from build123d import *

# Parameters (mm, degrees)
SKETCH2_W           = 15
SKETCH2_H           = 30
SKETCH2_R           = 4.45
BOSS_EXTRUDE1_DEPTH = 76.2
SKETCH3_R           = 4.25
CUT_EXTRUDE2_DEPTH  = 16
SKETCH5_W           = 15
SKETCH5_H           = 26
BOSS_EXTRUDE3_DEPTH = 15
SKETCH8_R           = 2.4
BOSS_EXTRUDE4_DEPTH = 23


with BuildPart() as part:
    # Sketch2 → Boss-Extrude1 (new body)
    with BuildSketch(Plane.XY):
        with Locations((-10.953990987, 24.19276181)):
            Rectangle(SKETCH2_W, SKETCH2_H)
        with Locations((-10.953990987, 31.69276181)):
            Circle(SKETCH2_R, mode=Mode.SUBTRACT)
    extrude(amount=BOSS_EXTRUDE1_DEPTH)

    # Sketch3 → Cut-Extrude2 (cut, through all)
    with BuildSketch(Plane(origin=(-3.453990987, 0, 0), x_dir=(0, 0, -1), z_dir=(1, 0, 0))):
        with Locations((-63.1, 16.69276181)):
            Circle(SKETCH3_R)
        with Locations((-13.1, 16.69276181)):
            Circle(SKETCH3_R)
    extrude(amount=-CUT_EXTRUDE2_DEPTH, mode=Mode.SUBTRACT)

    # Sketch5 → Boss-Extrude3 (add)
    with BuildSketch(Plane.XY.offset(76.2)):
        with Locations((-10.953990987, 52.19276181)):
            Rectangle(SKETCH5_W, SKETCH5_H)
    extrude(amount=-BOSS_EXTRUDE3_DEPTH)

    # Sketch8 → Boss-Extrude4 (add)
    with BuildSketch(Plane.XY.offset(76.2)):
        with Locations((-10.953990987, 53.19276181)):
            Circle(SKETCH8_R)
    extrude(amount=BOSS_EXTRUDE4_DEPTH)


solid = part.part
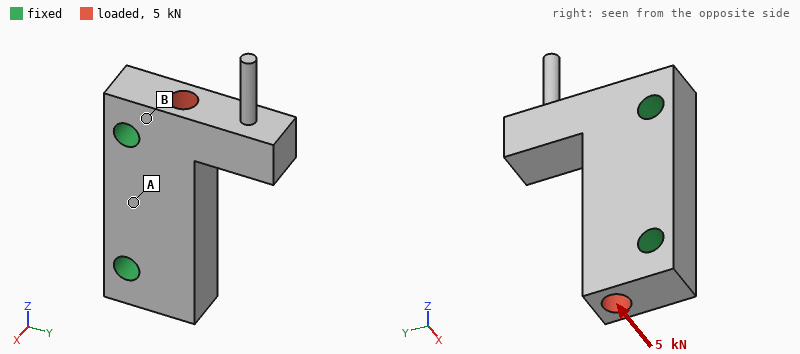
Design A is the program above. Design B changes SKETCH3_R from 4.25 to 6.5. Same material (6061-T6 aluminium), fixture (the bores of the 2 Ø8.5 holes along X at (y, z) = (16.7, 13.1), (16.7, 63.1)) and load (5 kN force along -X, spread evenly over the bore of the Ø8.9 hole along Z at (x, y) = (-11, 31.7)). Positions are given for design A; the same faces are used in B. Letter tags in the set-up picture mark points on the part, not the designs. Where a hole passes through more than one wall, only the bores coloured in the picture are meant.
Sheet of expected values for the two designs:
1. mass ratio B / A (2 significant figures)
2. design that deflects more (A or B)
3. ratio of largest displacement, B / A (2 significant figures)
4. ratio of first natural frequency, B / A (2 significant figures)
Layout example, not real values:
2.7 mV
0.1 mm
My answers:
0.93
A
0.69
1.0
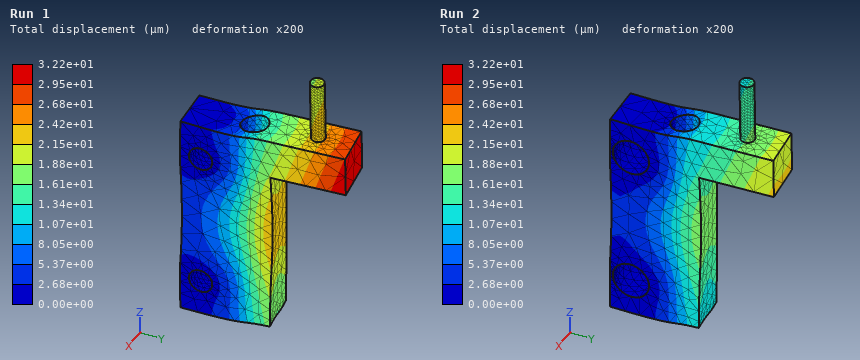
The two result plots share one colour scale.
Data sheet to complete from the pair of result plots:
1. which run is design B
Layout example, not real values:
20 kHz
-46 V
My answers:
Run 2
